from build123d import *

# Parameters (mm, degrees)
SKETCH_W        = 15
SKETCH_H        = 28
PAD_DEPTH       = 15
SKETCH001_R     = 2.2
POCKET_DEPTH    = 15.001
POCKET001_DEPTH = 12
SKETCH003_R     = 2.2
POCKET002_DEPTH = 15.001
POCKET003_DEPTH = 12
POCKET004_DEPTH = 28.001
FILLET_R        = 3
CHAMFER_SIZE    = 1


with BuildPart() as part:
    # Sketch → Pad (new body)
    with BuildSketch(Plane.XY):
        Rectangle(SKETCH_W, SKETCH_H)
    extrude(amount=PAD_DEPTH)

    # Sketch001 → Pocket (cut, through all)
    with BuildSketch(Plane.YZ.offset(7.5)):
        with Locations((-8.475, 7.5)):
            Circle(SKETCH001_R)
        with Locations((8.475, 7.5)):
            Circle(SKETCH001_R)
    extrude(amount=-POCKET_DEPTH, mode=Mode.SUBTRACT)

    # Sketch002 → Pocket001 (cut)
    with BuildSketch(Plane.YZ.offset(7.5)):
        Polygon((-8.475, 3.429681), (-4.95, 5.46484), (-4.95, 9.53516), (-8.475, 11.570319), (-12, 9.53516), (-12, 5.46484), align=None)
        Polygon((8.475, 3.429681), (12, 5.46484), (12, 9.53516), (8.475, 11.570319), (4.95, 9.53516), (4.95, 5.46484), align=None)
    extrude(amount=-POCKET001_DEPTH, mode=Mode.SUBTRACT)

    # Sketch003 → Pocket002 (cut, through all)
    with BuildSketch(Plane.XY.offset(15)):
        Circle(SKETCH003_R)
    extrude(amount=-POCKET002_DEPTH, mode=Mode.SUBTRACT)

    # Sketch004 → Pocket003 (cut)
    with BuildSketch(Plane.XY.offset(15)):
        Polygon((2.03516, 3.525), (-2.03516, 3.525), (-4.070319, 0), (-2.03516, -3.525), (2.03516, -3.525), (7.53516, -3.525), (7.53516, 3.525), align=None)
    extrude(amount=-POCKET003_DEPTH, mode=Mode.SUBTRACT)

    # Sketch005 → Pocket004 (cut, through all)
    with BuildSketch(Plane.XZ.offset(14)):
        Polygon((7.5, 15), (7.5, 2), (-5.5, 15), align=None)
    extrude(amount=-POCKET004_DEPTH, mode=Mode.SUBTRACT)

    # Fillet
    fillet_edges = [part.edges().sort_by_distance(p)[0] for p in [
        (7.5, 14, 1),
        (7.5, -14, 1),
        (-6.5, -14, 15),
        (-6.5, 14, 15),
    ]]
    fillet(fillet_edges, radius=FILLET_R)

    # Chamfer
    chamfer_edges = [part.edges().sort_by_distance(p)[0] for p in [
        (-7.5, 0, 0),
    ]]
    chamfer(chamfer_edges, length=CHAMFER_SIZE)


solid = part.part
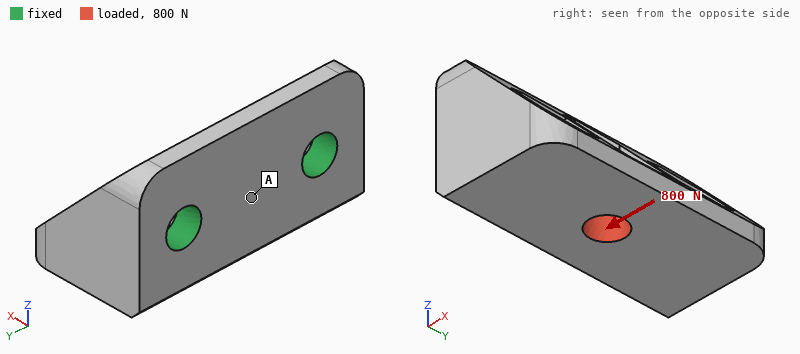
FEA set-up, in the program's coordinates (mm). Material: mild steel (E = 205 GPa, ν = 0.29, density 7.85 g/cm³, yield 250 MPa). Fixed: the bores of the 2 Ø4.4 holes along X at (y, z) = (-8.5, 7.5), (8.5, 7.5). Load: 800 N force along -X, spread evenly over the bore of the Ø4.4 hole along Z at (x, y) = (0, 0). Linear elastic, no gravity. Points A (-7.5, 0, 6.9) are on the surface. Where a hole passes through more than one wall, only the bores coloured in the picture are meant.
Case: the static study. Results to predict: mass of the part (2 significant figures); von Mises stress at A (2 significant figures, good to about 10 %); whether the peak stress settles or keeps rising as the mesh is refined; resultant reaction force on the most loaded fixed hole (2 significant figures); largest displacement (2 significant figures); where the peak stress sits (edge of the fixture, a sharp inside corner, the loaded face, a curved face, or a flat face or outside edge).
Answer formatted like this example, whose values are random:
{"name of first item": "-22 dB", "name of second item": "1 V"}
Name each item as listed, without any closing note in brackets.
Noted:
{"mass of the part": "23 g", "von Mises stress at A": "10 MPa", "whether the peak stress settles or keeps rising as the mesh is refined": "keeps rising", "resultant reaction force on the most loaded fixed hole": "420 N", "largest displacement": "6.2 µm", "where the peak stress sits": "edge of the fixture"}
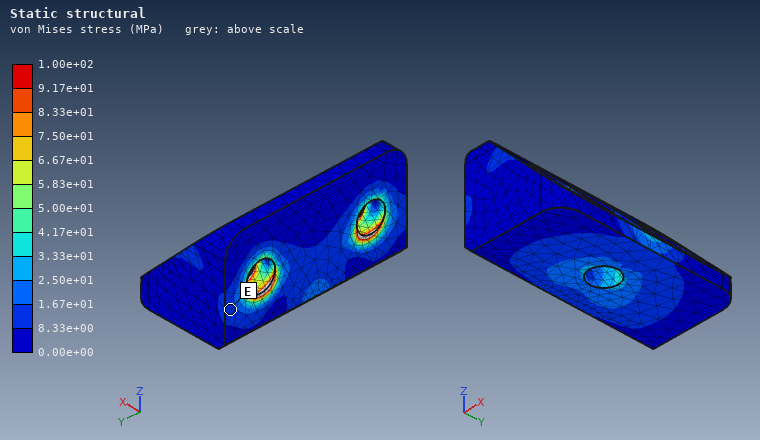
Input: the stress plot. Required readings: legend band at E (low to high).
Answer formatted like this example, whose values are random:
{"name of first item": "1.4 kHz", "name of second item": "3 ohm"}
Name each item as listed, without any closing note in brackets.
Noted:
{"legend band at E": "8.33e+00 to 1.67e+01 MPa"}
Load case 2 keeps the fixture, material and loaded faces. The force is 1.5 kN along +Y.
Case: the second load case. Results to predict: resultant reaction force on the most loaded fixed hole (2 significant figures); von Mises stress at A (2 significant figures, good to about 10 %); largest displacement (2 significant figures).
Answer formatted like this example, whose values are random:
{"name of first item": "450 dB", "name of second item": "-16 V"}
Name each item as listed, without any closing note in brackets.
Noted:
{"resultant reaction force on the most loaded fixed hole": "960 N", "von Mises stress at A": "8.8 MPa", "largest displacement": "4.0 µm"}
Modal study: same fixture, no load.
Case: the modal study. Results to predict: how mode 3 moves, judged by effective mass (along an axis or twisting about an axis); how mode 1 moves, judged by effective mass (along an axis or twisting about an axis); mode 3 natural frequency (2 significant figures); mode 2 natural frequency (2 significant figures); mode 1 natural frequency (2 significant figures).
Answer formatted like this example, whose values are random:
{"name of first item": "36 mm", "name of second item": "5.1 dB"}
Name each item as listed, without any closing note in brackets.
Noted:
{"how mode 3 moves, judged by effective mass": "along Y", "how mode 1 moves, judged by effective mass": "along Z", "mode 3 natural frequency": "35 kHz", "mode 2 natural frequency": "23 kHz", "mode 1 natural frequency": "17 kHz"}
